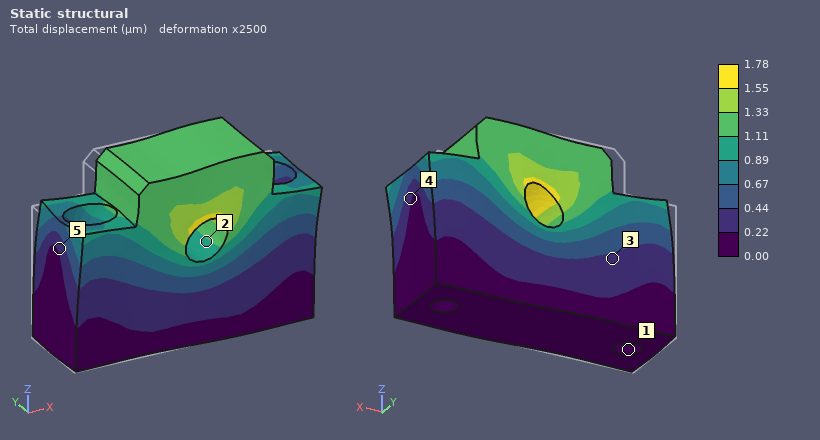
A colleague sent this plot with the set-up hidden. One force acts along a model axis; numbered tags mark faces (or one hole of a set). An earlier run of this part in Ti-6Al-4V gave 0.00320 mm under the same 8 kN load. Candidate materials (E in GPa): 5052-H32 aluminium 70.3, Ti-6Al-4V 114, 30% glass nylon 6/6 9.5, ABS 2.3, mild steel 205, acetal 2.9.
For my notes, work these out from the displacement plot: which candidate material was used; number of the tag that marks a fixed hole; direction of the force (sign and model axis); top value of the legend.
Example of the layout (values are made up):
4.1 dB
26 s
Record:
mild steel
1
+X
1.78 µm
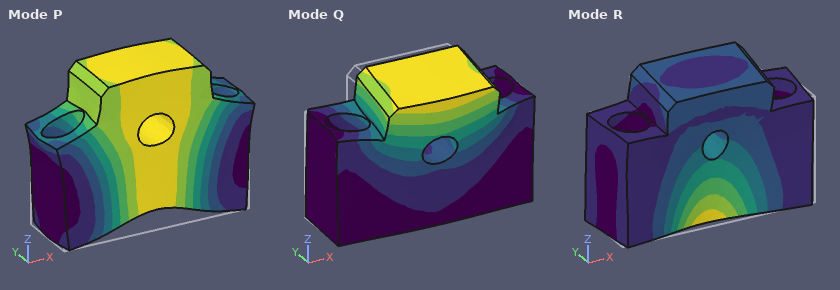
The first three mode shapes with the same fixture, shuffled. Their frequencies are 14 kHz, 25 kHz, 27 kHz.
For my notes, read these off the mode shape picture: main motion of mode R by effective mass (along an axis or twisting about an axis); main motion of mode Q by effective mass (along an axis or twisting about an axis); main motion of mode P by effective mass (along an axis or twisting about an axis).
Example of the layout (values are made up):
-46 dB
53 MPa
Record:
along Y
along Y
along Z
